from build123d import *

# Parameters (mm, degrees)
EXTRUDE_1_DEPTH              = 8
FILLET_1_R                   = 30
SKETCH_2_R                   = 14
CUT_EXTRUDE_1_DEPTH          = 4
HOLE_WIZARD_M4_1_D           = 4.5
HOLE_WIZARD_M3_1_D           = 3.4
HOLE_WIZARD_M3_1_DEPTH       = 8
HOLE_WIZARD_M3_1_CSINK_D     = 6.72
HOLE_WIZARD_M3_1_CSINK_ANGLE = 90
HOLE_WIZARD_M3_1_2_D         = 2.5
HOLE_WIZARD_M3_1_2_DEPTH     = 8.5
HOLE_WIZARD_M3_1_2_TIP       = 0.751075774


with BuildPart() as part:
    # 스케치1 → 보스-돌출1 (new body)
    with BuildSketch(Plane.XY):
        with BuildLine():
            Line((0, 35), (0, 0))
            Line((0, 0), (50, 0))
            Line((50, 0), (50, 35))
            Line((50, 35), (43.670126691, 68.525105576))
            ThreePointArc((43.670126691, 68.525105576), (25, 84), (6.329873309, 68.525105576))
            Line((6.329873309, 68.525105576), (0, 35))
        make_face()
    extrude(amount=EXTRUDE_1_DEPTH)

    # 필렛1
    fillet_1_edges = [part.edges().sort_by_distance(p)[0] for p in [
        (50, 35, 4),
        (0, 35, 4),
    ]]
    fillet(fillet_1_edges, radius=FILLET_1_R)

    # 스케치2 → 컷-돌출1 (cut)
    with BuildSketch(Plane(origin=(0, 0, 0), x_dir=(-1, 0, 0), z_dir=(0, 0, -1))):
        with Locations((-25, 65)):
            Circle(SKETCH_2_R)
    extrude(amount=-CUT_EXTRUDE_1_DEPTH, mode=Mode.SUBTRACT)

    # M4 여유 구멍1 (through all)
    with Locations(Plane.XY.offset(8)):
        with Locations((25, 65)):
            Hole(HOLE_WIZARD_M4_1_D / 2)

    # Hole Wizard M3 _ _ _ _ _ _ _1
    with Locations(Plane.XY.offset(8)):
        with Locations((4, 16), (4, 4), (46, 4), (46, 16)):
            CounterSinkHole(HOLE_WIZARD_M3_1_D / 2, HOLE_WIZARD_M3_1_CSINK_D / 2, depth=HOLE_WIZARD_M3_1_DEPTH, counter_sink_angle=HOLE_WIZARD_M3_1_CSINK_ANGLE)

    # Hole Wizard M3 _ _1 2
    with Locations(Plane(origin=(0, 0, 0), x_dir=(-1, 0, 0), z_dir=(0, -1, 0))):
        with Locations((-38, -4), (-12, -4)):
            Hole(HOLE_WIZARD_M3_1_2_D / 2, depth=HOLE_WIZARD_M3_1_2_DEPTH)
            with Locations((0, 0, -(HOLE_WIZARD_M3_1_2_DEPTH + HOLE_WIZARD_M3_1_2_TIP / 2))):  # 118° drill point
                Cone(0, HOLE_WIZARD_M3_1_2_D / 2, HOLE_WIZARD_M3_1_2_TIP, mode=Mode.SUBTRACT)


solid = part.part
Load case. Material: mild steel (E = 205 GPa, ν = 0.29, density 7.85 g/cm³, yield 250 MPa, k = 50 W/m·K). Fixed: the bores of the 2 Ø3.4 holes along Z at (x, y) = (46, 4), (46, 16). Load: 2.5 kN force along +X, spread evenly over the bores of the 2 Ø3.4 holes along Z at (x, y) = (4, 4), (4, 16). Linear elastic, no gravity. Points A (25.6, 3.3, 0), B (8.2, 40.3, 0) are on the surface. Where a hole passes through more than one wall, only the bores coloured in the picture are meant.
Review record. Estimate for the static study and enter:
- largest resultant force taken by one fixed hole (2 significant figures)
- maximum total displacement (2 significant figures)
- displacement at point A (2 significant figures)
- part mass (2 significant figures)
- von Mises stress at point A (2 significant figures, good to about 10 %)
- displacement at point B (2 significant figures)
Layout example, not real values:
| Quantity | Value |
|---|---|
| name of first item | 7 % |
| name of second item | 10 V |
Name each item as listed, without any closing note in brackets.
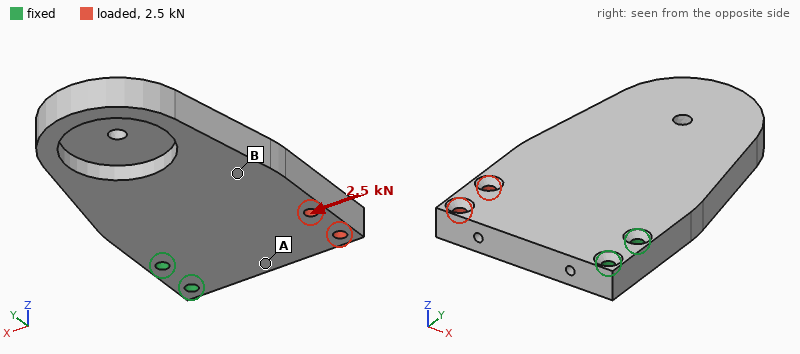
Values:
| Quantity | Value |
|---|---|
| largest resultant force taken by one fixed hole | 1.3 kN |
| maximum total displacement | 9.2 µm |
| displacement at point A | 2.8 µm |
| part mass | 210 g |
| von Mises stress at point A | 22 MPa |
| displacement at point B | 4.5 µm |
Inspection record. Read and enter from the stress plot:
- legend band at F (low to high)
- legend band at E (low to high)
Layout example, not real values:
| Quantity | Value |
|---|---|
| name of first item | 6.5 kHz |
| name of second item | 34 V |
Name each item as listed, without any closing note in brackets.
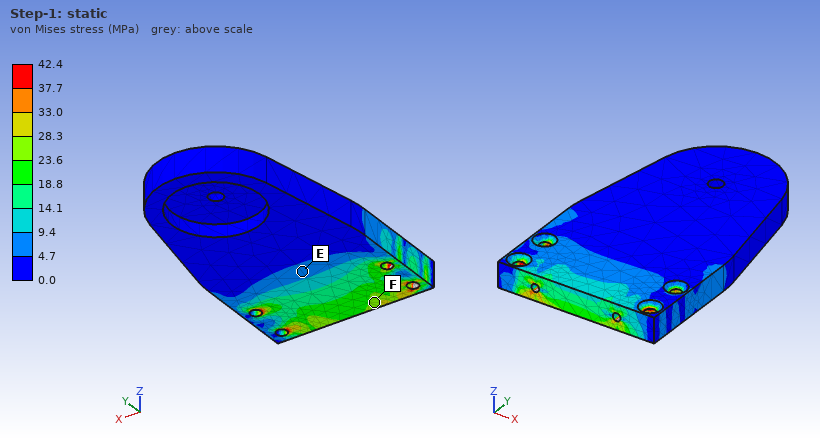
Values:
| Quantity | Value |
|---|---|
| legend band at F | 23.6 to 28.3 MPa |
| legend band at E | 4.7 to 9.4 MPa |
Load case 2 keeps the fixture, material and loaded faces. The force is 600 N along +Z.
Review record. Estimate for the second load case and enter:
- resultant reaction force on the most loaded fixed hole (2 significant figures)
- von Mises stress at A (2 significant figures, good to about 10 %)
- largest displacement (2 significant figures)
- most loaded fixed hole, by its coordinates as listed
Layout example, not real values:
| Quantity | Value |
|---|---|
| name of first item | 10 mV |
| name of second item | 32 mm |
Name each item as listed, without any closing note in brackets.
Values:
| Quantity | Value |
|---|---|
| resultant reaction force on the most loaded fixed hole | 340 N |
| von Mises stress at A | 36 MPa |
| largest displacement | 78 µm |
| most loaded fixed hole, by its coordinates as listed | (46, 16) |
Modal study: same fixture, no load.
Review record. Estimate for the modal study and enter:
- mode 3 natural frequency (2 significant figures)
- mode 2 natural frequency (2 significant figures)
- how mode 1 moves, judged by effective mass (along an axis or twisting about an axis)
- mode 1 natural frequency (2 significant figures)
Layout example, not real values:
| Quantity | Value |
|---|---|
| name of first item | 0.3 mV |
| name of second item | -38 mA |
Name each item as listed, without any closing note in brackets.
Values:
| Quantity | Value |
|---|---|
| mode 3 natural frequency | 2700 Hz |
| mode 2 natural frequency | 2500 Hz |
| how mode 1 moves, judged by effective mass | along Z |
| mode 1 natural frequency | 1200 Hz |
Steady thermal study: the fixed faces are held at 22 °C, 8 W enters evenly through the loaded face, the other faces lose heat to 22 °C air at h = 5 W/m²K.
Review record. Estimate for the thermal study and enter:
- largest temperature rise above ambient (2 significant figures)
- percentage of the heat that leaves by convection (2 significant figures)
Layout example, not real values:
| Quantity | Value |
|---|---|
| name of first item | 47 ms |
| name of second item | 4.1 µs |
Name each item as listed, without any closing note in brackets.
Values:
| Quantity | Value |
|---|---|
| largest temperature rise above ambient | 32 K |
| percentage of the heat that leaves by convection | 7.6 % |
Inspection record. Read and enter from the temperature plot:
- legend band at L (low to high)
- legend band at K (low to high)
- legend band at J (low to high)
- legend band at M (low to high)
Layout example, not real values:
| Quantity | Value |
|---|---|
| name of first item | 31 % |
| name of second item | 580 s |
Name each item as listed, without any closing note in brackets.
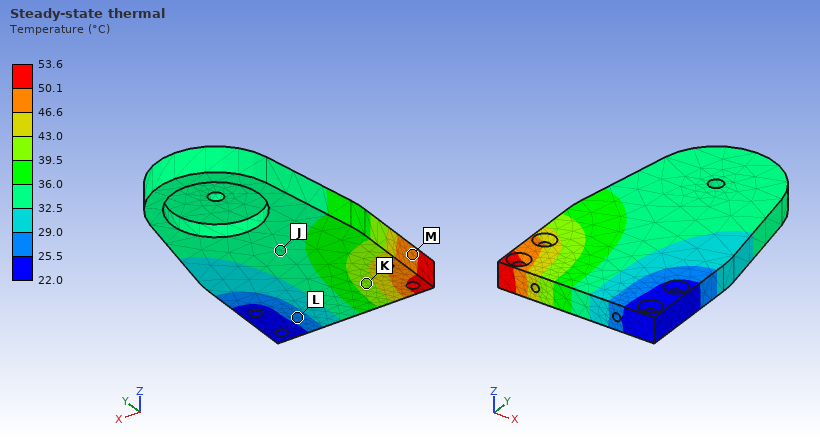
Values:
| Quantity | Value |
|---|---|
| legend band at L | 25.5 to 29.0 °C |
| legend band at K | 39.5 to 43.0 °C |
| legend band at J | 32.5 to 36.0 °C |
| legend band at M | 46.6 to 50.1 °C |
